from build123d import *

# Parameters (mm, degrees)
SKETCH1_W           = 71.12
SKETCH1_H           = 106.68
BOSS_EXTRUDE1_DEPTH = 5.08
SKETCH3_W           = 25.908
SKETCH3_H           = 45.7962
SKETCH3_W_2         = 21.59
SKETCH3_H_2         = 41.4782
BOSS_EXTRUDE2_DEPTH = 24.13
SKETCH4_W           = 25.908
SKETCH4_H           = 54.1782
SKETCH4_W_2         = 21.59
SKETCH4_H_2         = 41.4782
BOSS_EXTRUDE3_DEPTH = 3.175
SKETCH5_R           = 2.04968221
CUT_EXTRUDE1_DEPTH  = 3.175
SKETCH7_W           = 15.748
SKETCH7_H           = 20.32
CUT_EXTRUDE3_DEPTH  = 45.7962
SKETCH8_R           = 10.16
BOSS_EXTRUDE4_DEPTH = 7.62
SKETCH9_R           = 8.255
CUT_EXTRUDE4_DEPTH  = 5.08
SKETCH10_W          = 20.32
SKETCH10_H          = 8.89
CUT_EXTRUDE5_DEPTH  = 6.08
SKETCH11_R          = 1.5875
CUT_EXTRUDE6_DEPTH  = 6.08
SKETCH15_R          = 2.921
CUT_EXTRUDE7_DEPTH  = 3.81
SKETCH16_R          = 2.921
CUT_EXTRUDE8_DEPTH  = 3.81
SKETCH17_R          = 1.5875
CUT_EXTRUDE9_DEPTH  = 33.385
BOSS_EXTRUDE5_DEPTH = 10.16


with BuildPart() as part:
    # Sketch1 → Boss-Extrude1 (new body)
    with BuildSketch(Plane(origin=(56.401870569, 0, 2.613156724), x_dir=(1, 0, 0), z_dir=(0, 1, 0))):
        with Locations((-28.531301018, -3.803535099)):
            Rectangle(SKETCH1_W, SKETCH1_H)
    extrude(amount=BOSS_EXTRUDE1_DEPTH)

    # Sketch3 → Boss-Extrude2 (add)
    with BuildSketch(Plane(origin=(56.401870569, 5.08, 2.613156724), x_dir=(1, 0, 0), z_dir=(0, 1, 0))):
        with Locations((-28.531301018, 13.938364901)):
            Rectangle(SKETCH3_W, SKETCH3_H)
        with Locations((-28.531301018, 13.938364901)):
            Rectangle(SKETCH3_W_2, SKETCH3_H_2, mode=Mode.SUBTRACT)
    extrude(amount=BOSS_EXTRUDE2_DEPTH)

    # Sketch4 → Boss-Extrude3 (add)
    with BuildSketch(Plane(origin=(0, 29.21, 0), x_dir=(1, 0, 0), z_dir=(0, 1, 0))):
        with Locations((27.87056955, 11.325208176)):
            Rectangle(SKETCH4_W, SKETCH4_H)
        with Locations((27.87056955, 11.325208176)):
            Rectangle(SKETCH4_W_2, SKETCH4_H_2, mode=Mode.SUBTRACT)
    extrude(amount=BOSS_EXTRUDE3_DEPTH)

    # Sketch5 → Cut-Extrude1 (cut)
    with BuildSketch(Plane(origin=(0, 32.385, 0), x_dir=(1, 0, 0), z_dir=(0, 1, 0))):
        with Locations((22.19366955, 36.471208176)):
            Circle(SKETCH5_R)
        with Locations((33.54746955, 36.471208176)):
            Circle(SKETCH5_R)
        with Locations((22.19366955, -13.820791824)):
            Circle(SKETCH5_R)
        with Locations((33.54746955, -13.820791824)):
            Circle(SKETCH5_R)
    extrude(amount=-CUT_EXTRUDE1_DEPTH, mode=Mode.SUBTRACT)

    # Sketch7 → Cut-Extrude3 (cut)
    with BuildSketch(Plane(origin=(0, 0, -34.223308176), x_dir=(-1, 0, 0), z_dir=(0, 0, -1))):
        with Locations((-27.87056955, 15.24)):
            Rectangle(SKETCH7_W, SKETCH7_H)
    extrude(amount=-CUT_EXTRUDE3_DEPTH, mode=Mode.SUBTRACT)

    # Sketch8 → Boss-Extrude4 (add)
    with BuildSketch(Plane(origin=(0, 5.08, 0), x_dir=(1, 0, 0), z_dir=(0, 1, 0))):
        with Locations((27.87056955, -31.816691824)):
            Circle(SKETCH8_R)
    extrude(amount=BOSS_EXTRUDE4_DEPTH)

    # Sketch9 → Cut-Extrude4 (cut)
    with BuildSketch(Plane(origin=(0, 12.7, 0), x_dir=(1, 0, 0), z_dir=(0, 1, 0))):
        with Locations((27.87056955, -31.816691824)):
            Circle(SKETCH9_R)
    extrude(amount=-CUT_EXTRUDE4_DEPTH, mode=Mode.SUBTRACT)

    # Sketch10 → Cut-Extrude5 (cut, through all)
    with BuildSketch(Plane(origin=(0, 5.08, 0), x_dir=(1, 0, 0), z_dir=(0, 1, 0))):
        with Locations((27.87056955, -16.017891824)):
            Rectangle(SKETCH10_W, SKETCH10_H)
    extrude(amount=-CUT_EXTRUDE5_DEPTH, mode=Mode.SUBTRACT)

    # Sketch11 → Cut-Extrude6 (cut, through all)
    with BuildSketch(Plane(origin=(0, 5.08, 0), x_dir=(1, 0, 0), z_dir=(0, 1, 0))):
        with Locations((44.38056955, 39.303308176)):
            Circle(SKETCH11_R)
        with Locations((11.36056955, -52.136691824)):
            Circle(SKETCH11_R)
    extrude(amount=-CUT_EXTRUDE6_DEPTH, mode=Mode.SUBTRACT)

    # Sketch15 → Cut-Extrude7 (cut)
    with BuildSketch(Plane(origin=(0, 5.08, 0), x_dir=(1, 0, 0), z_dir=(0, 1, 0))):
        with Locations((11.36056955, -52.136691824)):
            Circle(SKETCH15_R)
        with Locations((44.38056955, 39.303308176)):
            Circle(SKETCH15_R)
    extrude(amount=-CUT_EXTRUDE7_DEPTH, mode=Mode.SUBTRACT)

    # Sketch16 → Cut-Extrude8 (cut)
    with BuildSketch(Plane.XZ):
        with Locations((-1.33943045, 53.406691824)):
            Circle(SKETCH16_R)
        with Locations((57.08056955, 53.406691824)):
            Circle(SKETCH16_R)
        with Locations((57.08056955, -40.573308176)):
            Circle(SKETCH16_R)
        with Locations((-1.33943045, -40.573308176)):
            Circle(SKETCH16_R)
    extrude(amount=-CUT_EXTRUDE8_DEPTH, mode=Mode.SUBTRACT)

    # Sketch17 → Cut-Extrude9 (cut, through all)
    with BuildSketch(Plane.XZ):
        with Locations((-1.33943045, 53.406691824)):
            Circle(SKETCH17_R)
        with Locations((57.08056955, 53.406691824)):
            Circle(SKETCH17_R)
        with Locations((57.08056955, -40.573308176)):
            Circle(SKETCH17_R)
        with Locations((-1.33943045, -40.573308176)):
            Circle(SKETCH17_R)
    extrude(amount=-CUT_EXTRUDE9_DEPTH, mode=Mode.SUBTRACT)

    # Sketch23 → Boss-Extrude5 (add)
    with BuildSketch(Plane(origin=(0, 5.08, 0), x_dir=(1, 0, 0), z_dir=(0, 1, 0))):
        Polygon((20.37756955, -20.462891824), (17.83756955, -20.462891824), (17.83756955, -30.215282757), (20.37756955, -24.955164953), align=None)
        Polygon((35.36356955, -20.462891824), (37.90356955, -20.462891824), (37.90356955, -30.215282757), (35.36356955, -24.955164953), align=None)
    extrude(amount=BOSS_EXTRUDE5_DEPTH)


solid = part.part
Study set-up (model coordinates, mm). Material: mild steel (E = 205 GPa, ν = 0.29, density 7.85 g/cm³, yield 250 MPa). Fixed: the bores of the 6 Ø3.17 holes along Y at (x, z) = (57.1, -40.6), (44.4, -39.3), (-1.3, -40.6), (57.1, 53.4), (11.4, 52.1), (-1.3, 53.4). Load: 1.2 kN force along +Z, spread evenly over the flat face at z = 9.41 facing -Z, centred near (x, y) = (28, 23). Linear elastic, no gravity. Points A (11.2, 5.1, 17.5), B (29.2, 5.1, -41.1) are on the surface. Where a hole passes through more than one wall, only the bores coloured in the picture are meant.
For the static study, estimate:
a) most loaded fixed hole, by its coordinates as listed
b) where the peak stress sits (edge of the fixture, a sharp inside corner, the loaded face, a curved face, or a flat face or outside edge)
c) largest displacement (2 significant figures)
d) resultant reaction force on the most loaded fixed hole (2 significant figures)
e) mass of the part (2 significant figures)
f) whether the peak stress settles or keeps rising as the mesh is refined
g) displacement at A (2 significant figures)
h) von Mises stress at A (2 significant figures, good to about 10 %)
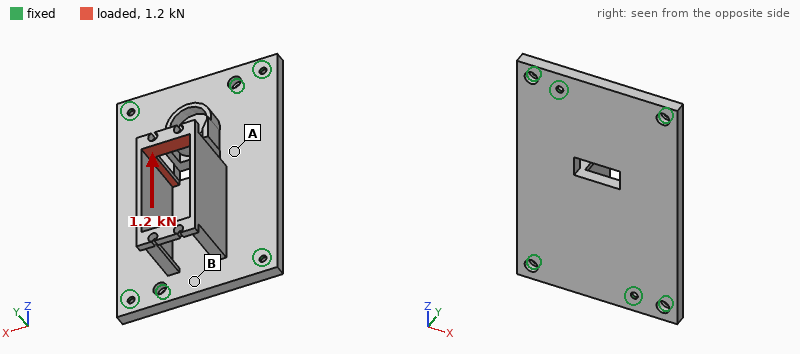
(11.4, 52.1)
a sharp inside corner
56 µm
780 N
360 g
keeps rising
21 µm
32 MPa
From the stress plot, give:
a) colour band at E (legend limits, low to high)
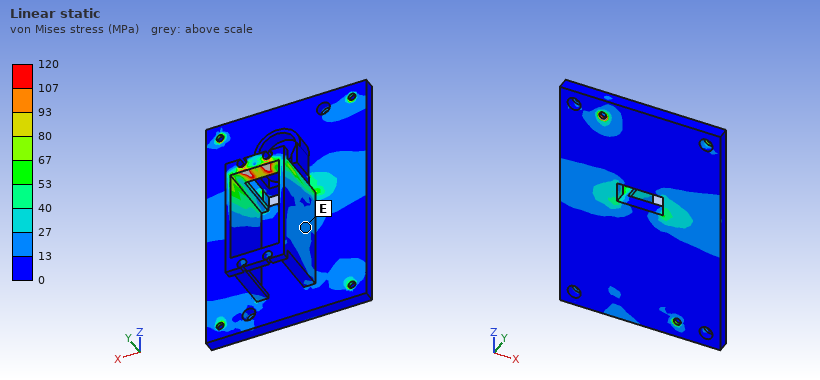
13 to 27 MPa
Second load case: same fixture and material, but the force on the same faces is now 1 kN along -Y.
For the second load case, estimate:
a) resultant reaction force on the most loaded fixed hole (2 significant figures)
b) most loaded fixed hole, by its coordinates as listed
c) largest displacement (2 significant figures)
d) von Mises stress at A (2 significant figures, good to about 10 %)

1.2 kN
(11.4, 52.1)
69 µm
52 MPa
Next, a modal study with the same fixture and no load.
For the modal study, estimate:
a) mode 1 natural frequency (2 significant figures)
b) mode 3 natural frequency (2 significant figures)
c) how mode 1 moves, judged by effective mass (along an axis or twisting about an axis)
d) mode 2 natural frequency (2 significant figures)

1900 Hz
4600 Hz
along Y
2800 Hz
